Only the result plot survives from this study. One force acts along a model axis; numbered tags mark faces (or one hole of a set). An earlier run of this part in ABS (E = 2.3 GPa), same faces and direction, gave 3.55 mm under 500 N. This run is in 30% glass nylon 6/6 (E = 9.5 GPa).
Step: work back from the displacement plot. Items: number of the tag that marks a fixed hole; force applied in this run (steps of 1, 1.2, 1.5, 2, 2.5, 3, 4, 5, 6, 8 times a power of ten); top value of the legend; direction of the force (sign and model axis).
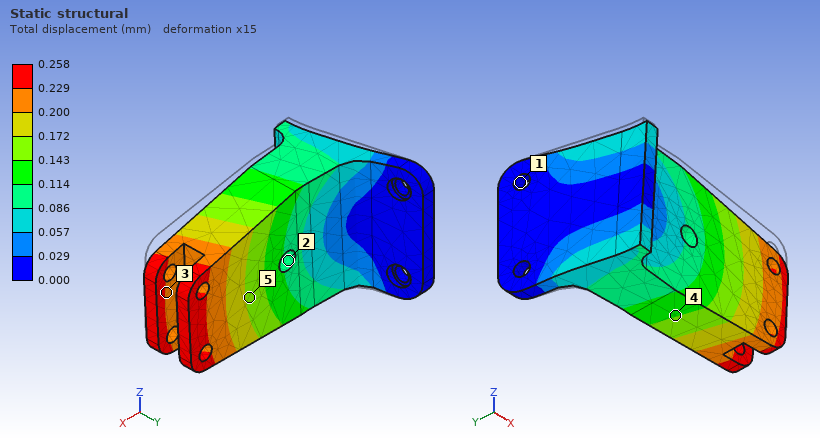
1
150 N
0.258 mm
-Z
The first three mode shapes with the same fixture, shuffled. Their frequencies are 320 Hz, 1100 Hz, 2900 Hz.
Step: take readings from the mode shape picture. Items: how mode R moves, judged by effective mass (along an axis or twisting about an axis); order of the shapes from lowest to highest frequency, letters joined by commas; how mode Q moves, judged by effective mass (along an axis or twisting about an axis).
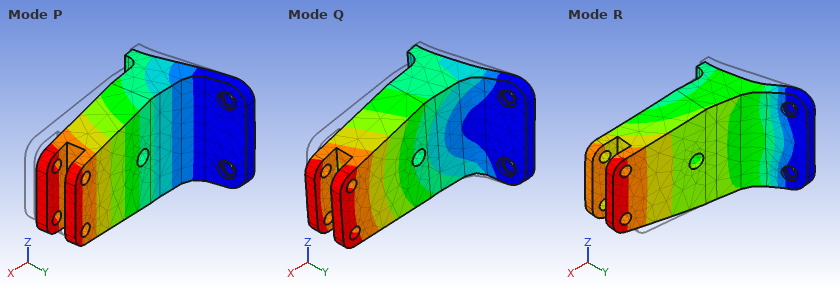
along X
P, Q, R
along Z
